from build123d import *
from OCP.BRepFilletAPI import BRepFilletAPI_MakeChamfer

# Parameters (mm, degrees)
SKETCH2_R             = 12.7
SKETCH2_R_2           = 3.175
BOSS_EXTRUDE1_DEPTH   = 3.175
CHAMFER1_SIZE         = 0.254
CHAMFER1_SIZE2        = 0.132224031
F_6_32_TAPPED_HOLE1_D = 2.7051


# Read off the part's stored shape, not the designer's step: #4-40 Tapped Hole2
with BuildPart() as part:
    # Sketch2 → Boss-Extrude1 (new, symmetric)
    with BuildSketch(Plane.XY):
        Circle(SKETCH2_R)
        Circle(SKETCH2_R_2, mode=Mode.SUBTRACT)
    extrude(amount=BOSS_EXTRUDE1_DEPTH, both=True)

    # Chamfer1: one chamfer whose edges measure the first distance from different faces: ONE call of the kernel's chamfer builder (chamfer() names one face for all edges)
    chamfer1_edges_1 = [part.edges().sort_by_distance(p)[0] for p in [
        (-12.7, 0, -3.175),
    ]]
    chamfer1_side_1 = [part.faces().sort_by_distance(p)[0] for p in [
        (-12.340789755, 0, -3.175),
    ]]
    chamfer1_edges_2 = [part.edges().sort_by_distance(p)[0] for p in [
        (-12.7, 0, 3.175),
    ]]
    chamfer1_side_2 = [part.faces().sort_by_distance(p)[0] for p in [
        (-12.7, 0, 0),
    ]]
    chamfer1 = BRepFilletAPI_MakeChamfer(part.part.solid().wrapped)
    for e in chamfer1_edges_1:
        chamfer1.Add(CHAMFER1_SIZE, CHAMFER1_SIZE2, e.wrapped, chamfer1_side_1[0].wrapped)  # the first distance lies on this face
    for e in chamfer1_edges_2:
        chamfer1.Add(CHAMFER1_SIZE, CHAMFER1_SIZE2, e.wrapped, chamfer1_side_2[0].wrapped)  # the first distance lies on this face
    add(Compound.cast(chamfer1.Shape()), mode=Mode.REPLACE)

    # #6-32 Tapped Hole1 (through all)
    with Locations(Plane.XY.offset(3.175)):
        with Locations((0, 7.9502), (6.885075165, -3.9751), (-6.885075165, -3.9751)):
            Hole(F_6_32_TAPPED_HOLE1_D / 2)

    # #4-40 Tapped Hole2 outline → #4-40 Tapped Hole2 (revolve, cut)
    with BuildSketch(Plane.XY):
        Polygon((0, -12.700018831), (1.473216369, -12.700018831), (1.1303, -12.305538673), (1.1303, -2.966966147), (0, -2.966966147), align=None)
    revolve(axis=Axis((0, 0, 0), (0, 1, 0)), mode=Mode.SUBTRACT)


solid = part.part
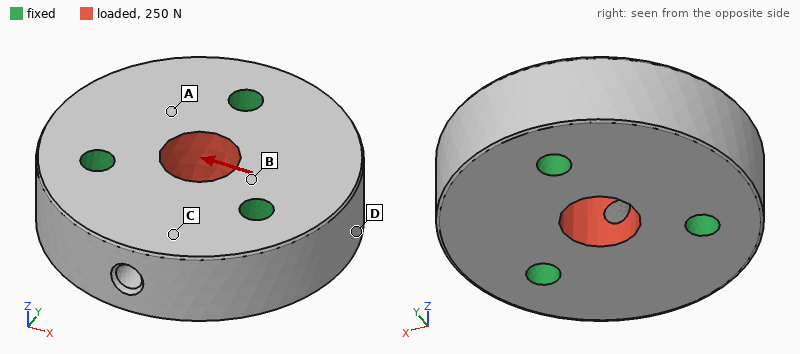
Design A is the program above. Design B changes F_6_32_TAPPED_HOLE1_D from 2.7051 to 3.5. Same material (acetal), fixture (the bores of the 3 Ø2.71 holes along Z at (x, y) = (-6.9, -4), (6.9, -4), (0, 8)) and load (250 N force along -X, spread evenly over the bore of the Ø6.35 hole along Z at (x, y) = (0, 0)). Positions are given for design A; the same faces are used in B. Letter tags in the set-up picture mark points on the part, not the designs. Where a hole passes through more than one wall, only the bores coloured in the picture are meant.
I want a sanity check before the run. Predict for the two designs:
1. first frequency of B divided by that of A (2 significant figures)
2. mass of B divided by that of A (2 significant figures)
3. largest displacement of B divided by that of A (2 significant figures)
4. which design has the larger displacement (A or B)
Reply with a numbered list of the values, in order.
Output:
1. 1.1
2. 0.97
3. 0.91
4. A
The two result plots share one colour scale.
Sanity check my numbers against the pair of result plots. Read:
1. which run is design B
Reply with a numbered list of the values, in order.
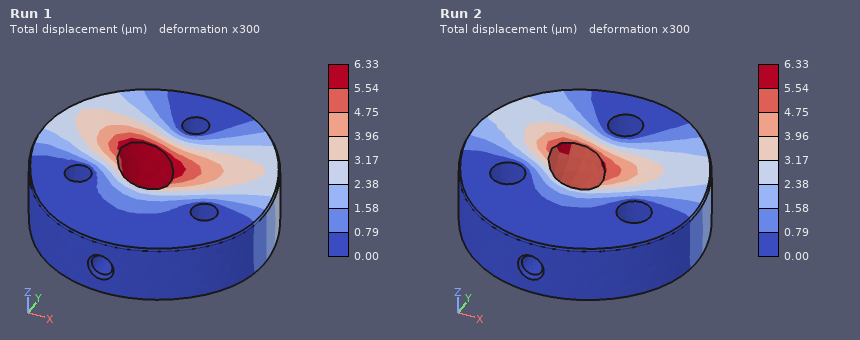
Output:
1. Run 2
